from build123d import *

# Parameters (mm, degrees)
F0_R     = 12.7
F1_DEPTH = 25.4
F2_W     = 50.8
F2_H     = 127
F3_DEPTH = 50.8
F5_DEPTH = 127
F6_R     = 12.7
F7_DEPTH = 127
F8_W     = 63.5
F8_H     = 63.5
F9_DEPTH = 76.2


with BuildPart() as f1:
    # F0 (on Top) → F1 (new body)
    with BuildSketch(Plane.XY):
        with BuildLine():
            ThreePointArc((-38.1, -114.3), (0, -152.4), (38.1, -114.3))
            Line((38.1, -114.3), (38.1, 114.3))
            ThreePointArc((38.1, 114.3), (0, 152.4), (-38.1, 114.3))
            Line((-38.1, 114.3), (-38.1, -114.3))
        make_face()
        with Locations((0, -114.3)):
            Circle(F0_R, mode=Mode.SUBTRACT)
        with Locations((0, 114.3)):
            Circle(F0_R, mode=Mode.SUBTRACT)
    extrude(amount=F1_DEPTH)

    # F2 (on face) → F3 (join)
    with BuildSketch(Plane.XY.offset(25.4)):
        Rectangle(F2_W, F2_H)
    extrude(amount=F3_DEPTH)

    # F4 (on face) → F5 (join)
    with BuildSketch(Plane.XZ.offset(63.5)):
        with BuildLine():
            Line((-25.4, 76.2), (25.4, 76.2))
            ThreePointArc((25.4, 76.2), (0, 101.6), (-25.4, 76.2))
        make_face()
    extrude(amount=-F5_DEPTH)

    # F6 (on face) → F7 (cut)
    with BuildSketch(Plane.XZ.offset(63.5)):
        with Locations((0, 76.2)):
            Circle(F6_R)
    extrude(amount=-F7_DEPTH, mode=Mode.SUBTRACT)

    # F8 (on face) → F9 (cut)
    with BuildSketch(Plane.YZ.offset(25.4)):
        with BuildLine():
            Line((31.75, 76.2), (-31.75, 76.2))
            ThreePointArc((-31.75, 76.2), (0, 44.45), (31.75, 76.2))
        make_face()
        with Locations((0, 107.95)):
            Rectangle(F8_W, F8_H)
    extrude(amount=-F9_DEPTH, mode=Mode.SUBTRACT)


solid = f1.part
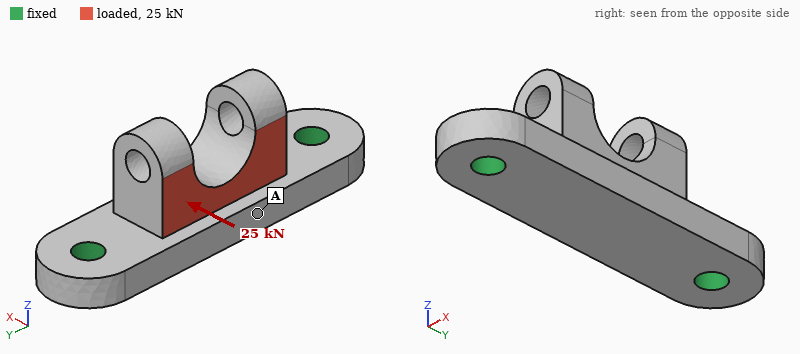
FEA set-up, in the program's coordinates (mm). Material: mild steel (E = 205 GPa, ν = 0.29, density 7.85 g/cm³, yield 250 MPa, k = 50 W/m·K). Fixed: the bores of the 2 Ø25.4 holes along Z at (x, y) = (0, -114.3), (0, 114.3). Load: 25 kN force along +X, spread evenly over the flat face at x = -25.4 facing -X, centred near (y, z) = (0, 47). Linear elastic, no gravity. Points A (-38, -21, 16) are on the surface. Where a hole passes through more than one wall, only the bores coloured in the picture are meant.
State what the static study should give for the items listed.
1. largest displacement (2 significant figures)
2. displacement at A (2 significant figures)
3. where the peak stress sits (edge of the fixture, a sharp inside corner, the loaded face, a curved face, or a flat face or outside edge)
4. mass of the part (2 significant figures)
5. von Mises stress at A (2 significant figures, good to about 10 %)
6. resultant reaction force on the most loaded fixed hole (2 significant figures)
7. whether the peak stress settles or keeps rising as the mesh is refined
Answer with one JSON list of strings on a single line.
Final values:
["85 µm", "34 µm", "edge of the fixture", "6.4 kg", "14 MPa", "13 kN", "keeps rising"]
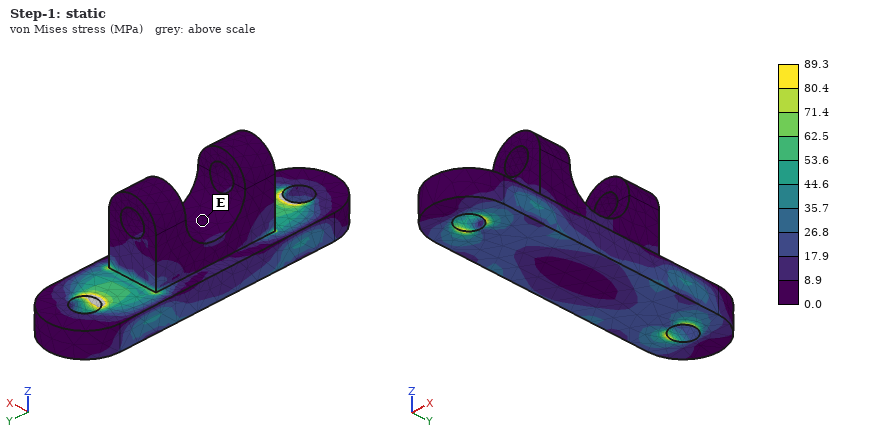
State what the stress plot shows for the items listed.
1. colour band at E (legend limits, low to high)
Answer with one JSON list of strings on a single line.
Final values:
["0.0 to 8.9 MPa"]
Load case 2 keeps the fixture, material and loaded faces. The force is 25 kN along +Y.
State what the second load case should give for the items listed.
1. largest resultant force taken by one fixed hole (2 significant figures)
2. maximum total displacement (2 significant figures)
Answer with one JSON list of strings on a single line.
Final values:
["14 kN", "15 µm"]
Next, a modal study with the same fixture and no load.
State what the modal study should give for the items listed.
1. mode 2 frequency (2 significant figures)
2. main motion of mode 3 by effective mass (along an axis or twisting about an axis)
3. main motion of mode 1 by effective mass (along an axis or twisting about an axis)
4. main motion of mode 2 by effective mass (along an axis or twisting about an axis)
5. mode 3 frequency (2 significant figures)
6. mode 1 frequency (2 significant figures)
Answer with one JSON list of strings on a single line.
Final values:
["2500 Hz", "along X", "along X", "along Z", "4000 Hz", "2000 Hz"]
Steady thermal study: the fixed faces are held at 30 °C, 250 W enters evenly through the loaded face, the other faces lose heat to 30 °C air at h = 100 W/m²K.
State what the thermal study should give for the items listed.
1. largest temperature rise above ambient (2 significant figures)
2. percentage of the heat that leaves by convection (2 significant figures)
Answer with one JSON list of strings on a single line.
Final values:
["57 K", "69 %"]
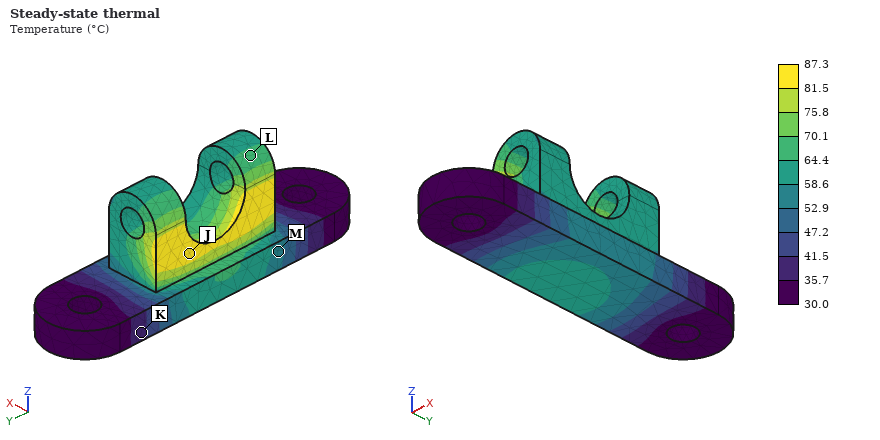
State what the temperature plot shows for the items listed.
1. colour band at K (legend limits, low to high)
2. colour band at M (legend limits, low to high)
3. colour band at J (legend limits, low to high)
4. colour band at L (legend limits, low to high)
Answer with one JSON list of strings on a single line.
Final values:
["35.7 to 41.5 °C", "52.9 to 58.6 °C", "81.5 to 87.3 °C", "64.4 to 70.1 °C"]
